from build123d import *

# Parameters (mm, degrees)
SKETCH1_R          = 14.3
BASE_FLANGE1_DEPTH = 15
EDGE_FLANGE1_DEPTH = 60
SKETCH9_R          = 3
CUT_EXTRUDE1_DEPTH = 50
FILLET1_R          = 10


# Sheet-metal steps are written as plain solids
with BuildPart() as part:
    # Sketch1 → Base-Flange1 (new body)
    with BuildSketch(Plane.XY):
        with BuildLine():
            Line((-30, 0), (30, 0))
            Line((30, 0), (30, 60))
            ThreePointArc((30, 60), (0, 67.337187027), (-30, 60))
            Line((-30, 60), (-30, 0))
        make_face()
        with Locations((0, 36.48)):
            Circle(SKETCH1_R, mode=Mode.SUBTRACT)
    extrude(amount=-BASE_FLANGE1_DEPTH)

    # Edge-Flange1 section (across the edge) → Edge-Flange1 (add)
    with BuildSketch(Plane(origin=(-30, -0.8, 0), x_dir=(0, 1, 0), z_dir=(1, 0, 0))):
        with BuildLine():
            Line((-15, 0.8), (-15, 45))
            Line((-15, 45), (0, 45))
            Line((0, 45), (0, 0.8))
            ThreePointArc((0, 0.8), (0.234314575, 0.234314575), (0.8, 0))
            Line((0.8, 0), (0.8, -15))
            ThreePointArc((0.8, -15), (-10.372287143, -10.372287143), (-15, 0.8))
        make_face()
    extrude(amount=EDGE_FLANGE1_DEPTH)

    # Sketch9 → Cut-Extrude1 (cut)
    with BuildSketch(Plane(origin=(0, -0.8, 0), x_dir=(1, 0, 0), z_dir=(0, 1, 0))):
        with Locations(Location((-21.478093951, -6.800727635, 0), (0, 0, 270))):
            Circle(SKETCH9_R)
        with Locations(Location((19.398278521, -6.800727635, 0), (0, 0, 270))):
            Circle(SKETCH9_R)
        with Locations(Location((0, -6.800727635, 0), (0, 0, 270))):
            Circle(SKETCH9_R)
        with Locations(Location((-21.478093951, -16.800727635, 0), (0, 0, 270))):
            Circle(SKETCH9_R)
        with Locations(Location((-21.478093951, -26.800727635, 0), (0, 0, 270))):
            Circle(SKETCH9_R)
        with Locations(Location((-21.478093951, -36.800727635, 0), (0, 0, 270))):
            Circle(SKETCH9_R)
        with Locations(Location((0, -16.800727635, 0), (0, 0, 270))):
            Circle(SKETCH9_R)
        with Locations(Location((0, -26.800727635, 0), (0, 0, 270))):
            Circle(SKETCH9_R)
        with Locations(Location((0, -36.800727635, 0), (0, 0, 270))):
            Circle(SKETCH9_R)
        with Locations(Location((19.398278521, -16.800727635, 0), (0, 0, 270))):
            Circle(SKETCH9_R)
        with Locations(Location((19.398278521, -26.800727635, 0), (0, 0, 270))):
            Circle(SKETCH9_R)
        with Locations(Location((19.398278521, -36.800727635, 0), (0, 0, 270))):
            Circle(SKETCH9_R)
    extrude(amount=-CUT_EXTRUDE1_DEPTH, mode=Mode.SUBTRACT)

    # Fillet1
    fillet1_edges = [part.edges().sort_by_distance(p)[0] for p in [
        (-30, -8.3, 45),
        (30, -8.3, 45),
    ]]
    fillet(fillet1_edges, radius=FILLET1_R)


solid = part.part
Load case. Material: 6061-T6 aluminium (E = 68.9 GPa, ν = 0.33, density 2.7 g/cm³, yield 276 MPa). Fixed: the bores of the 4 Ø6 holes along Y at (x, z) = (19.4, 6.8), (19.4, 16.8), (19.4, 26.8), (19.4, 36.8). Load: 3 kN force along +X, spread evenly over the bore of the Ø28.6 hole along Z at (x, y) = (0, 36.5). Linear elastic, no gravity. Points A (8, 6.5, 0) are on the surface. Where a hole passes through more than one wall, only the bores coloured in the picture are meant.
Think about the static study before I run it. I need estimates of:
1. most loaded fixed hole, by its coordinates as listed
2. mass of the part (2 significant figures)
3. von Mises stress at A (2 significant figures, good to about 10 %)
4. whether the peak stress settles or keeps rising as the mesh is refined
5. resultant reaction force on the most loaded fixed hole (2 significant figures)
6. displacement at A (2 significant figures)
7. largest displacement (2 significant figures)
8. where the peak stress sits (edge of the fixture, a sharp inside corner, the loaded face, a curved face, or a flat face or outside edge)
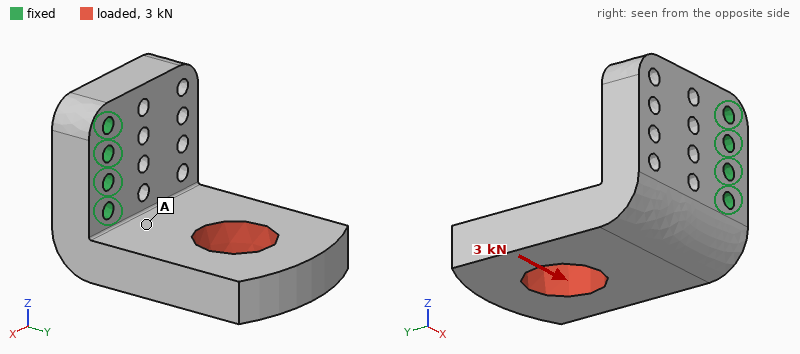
(19.4, 6.8)
260 g
26 MPa
keeps rising
4.0 kN
0.042 mm
0.21 mm
edge of the fixture
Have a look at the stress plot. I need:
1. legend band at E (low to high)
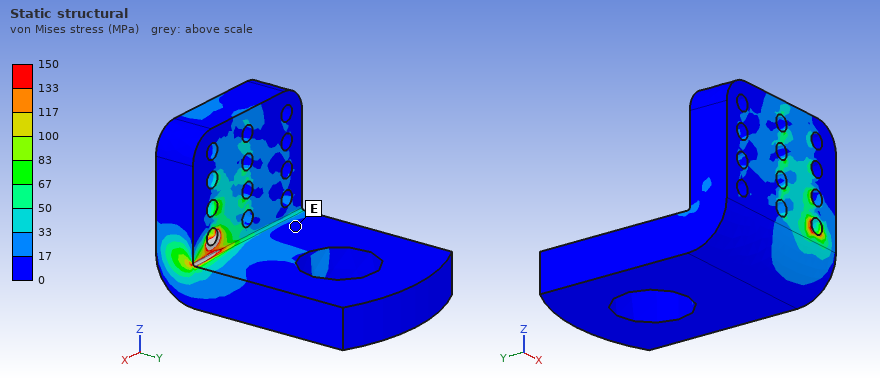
0 to 17 MPa
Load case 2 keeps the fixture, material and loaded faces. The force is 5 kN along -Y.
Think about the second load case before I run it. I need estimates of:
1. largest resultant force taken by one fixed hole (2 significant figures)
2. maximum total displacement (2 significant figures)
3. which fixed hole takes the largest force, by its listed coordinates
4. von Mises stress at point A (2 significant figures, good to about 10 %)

5.0 kN
0.18 mm
(19.4, 6.8)
12 MPa
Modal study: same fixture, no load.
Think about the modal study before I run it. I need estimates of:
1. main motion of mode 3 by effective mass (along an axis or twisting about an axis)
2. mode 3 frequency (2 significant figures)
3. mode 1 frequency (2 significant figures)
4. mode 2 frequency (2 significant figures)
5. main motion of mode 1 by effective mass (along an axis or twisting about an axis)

twisting about Y
4500 Hz
1500 Hz
2000 Hz
along Z
